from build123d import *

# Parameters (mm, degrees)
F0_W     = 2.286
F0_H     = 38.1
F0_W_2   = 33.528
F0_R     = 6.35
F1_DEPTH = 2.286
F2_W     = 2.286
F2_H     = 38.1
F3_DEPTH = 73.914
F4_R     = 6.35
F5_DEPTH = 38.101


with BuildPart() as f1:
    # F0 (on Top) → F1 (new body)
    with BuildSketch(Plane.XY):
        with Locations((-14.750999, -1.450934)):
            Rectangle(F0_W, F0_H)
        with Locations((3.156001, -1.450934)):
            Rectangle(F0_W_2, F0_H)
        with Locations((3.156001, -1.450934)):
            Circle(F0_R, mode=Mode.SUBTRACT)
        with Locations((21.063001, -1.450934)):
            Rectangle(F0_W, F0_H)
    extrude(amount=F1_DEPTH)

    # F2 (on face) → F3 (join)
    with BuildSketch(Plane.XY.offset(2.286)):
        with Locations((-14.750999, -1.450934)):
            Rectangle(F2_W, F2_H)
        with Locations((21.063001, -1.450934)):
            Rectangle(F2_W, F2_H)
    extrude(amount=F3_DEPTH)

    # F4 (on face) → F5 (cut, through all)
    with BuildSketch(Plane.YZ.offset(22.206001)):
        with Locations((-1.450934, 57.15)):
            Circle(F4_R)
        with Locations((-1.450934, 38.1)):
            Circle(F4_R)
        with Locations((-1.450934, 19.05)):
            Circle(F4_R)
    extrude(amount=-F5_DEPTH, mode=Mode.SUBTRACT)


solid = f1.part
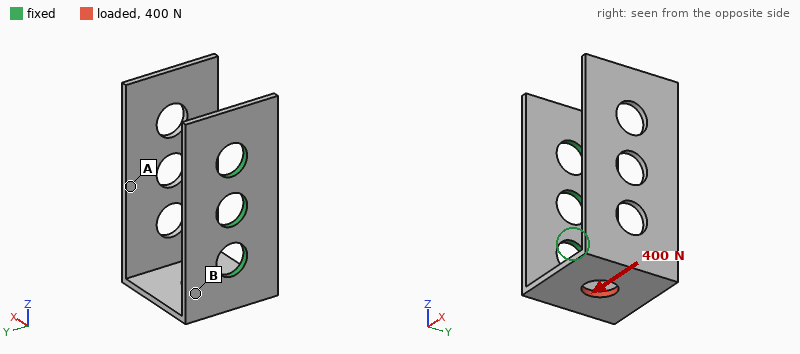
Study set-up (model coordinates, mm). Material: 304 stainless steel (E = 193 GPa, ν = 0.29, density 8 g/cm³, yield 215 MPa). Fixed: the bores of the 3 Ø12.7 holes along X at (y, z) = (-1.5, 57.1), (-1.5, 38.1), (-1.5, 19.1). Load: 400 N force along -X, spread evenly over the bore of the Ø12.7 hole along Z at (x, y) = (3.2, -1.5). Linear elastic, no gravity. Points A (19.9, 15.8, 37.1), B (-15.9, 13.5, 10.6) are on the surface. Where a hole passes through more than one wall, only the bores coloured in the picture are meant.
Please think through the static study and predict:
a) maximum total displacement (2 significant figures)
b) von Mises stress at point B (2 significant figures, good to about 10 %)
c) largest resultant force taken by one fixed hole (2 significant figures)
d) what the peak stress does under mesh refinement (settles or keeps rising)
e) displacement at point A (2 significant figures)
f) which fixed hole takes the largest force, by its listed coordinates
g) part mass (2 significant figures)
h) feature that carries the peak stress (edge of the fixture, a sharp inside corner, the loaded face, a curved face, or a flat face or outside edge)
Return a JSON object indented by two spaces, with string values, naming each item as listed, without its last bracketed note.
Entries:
{
  "maximum total displacement": "0.37 mm",
  "von Mises stress at point B": "65 MPa",
  "largest resultant force taken by one fixed hole": "420 N",
  "what the peak stress does under mesh refinement": "keeps rising",
  "displacement at point A": "0.22 mm",
  "which fixed hole takes the largest force, by its listed coordinates": "(-1.5, 19.1)",
  "part mass": "110 g",
  "feature that carries the peak stress": "edge of the fixture"
}
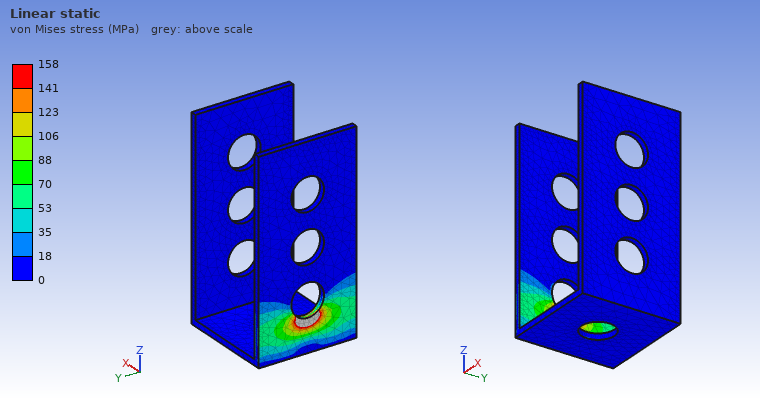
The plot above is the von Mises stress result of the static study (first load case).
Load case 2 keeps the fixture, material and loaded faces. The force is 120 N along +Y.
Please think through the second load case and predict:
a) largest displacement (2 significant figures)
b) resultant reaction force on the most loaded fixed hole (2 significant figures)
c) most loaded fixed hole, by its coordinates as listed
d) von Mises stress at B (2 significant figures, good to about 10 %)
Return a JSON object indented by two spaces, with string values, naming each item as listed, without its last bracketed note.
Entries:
{
  "largest displacement": "0.12 mm",
  "resultant reaction force on the most loaded fixed hole": "150 N",
  "most loaded fixed hole, by its coordinates as listed": "(-1.5, 19.1)",
  "von Mises stress at B": "20 MPa"
}
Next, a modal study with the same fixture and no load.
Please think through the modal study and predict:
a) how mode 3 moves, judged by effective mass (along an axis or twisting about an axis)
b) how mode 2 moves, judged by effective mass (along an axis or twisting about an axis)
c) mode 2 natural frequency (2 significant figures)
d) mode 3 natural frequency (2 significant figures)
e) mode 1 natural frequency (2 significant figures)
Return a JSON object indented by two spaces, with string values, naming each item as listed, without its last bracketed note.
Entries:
{
  "how mode 3 moves, judged by effective mass": "along Z",
  "how mode 2 moves, judged by effective mass": "along Y",
  "mode 2 natural frequency": "280 Hz",
  "mode 3 natural frequency": "510 Hz",
  "mode 1 natural frequency": "160 Hz"
}
